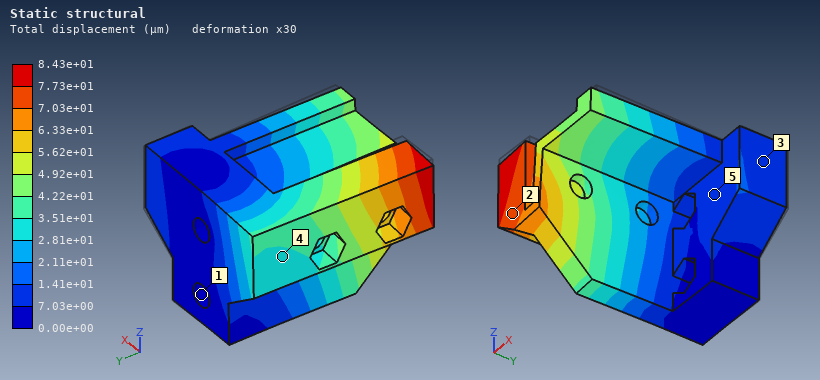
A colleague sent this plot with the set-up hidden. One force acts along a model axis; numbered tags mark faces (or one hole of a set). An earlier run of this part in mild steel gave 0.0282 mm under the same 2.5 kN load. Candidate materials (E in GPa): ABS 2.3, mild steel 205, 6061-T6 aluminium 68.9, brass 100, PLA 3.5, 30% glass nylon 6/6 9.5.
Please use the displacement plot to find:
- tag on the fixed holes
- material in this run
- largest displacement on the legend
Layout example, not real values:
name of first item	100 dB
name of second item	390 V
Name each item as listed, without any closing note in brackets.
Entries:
tag on the fixed holes	1
material in this run	6061-T6 aluminium
largest displacement on the legend	8.43e+01 µm
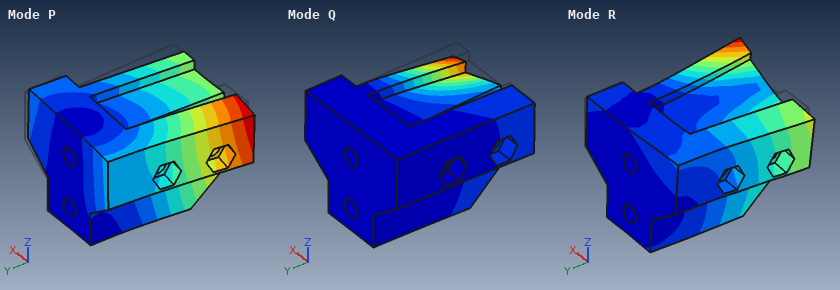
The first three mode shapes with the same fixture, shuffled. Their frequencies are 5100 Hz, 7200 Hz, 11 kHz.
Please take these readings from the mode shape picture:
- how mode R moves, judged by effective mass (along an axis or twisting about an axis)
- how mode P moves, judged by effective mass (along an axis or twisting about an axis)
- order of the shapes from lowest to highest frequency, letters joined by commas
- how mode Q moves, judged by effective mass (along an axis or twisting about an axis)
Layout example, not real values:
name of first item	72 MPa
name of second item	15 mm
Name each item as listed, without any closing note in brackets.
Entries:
how mode R moves, judged by effective mass	along Z
how mode P moves, judged by effective mass	along X
order of the shapes from lowest to highest frequency, letters joined by commas	P, Q, R
how mode Q moves, judged by effective mass	along Z
